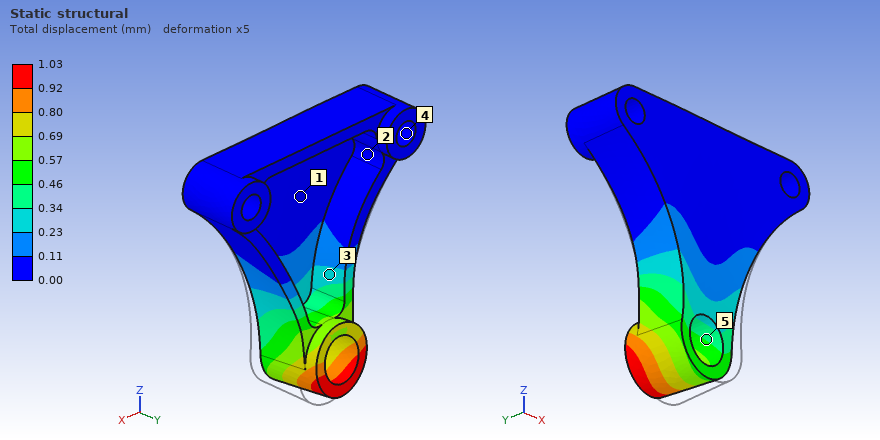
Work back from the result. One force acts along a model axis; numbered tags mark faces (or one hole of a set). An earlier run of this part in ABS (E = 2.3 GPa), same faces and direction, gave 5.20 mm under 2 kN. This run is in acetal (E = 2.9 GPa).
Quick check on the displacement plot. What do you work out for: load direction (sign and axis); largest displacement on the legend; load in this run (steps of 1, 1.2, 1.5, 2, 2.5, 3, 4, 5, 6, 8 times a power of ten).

-X
1.03 mm
500 N
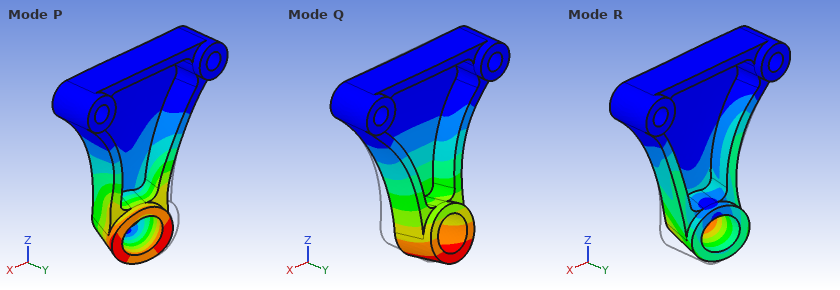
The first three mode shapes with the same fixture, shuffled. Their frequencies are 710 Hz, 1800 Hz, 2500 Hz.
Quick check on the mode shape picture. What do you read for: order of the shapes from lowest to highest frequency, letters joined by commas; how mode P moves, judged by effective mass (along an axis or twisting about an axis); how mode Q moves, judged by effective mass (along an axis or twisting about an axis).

Q, P, R
along X
along Y
